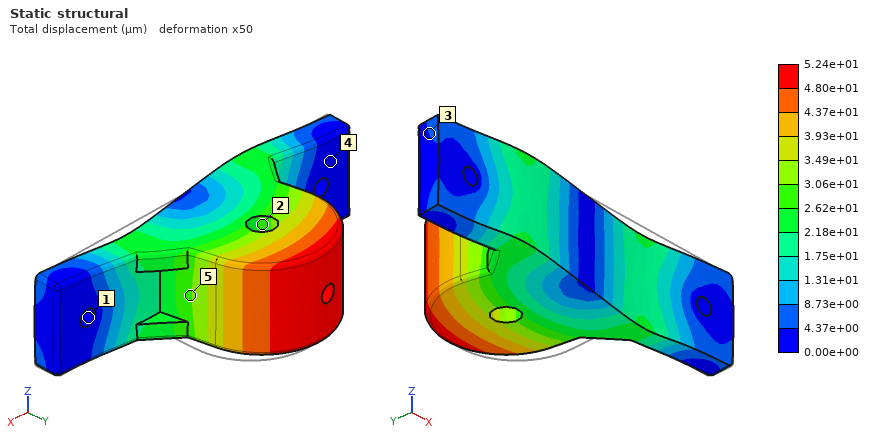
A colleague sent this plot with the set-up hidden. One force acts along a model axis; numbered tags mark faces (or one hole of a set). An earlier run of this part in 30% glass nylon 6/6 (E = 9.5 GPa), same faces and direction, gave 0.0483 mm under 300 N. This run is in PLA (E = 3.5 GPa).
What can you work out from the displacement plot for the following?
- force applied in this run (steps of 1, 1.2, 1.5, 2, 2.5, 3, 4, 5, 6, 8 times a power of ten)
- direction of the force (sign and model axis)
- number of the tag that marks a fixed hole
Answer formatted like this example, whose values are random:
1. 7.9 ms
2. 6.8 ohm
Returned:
1. 120 N
2. -X
3. 1
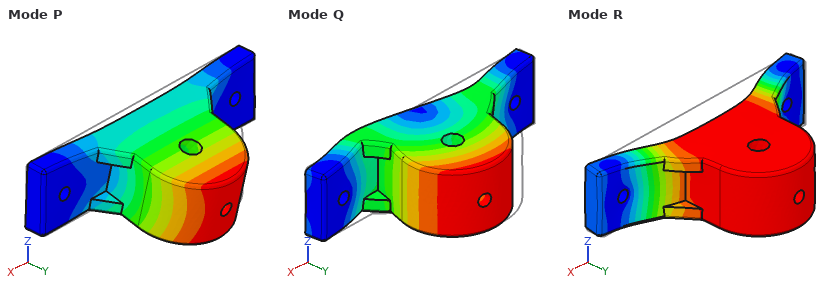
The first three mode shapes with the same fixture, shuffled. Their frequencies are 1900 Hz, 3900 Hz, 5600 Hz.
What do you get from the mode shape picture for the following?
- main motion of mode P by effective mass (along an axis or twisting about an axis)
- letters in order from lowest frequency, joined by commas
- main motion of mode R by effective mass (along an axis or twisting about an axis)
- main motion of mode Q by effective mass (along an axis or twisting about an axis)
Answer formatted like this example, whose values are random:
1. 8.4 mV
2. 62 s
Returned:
1. along Z
2. P, R, Q
3. along Y
4. along X
